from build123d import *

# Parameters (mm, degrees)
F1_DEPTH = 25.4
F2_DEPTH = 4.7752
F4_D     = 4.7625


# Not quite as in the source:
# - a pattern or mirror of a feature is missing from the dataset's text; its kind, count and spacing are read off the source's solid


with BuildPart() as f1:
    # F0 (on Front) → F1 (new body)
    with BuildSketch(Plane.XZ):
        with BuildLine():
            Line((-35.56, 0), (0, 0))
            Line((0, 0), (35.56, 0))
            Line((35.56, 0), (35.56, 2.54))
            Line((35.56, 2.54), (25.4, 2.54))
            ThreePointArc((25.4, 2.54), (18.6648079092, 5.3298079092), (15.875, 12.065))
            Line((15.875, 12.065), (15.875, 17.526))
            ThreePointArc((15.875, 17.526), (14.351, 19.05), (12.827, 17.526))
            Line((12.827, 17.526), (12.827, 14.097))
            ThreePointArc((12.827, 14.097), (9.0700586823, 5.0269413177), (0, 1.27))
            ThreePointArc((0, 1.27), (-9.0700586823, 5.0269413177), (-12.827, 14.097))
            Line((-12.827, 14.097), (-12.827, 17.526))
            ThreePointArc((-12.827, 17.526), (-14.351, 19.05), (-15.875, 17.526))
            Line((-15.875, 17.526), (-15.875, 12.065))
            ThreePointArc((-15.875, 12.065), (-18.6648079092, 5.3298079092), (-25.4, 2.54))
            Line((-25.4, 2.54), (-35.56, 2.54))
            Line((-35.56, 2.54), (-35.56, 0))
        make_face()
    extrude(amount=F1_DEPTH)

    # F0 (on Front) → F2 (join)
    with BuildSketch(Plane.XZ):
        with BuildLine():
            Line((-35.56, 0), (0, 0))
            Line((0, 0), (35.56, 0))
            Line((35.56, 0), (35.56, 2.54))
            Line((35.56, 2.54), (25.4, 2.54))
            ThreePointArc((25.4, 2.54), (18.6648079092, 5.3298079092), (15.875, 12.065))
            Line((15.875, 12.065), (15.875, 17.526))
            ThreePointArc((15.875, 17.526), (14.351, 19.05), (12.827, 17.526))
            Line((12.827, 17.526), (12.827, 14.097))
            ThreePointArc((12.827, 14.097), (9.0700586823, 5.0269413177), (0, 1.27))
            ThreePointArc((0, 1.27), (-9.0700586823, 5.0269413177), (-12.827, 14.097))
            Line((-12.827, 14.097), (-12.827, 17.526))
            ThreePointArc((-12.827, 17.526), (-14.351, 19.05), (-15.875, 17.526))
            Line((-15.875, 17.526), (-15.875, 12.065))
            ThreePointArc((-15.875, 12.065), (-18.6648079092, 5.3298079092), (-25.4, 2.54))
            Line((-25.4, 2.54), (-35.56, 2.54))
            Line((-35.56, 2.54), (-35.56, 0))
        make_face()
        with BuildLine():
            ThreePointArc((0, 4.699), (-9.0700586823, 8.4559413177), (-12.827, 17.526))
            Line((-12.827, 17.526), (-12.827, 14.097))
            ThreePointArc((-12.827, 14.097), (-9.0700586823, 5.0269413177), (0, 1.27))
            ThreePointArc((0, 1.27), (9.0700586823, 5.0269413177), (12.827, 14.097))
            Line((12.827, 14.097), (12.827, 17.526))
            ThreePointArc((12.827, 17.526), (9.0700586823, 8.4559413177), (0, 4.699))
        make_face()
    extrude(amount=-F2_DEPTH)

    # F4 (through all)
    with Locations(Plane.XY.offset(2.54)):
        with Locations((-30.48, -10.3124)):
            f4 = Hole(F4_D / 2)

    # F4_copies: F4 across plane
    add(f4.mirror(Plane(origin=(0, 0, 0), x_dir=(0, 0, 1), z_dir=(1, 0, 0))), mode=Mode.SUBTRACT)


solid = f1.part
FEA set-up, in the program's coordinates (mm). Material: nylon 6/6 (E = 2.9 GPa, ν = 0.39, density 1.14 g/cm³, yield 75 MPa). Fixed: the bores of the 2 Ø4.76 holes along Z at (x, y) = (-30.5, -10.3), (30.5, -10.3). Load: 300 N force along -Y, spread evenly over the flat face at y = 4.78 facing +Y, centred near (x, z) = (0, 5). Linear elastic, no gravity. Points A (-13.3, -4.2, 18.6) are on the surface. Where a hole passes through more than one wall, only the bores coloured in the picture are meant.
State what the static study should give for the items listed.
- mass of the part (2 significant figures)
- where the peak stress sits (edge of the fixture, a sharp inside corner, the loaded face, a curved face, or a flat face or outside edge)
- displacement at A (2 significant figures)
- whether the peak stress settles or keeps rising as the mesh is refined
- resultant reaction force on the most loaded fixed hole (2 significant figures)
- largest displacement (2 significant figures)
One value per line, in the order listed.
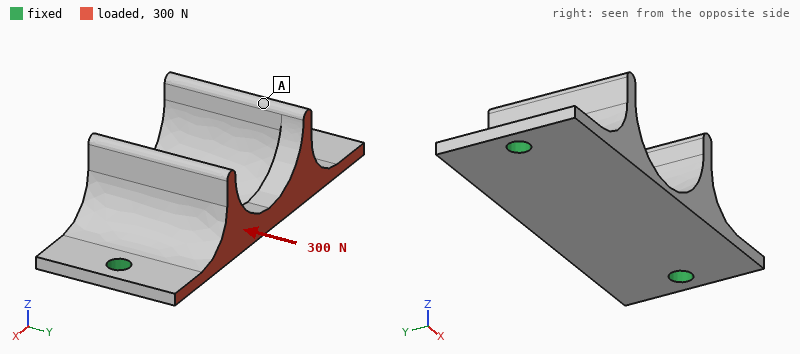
13 g
edge of the fixture
0.47 mm
keeps rising
150 N
0.58 mm
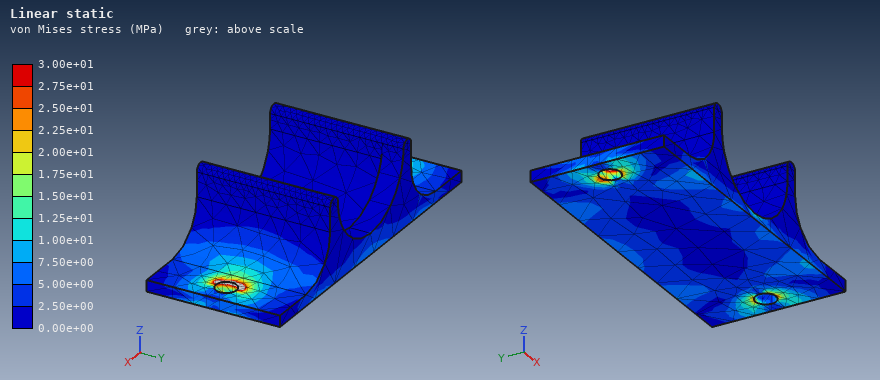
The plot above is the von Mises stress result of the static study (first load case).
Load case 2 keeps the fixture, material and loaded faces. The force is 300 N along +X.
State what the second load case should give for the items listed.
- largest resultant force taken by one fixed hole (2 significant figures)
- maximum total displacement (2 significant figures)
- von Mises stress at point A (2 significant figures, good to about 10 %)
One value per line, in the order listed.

170 N
0.10 mm
1.1 MPa
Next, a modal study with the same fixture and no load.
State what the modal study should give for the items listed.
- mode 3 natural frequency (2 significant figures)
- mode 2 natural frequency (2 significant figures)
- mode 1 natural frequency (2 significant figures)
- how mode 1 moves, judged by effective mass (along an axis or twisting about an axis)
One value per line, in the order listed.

2000 Hz
970 Hz
890 Hz
along Z
